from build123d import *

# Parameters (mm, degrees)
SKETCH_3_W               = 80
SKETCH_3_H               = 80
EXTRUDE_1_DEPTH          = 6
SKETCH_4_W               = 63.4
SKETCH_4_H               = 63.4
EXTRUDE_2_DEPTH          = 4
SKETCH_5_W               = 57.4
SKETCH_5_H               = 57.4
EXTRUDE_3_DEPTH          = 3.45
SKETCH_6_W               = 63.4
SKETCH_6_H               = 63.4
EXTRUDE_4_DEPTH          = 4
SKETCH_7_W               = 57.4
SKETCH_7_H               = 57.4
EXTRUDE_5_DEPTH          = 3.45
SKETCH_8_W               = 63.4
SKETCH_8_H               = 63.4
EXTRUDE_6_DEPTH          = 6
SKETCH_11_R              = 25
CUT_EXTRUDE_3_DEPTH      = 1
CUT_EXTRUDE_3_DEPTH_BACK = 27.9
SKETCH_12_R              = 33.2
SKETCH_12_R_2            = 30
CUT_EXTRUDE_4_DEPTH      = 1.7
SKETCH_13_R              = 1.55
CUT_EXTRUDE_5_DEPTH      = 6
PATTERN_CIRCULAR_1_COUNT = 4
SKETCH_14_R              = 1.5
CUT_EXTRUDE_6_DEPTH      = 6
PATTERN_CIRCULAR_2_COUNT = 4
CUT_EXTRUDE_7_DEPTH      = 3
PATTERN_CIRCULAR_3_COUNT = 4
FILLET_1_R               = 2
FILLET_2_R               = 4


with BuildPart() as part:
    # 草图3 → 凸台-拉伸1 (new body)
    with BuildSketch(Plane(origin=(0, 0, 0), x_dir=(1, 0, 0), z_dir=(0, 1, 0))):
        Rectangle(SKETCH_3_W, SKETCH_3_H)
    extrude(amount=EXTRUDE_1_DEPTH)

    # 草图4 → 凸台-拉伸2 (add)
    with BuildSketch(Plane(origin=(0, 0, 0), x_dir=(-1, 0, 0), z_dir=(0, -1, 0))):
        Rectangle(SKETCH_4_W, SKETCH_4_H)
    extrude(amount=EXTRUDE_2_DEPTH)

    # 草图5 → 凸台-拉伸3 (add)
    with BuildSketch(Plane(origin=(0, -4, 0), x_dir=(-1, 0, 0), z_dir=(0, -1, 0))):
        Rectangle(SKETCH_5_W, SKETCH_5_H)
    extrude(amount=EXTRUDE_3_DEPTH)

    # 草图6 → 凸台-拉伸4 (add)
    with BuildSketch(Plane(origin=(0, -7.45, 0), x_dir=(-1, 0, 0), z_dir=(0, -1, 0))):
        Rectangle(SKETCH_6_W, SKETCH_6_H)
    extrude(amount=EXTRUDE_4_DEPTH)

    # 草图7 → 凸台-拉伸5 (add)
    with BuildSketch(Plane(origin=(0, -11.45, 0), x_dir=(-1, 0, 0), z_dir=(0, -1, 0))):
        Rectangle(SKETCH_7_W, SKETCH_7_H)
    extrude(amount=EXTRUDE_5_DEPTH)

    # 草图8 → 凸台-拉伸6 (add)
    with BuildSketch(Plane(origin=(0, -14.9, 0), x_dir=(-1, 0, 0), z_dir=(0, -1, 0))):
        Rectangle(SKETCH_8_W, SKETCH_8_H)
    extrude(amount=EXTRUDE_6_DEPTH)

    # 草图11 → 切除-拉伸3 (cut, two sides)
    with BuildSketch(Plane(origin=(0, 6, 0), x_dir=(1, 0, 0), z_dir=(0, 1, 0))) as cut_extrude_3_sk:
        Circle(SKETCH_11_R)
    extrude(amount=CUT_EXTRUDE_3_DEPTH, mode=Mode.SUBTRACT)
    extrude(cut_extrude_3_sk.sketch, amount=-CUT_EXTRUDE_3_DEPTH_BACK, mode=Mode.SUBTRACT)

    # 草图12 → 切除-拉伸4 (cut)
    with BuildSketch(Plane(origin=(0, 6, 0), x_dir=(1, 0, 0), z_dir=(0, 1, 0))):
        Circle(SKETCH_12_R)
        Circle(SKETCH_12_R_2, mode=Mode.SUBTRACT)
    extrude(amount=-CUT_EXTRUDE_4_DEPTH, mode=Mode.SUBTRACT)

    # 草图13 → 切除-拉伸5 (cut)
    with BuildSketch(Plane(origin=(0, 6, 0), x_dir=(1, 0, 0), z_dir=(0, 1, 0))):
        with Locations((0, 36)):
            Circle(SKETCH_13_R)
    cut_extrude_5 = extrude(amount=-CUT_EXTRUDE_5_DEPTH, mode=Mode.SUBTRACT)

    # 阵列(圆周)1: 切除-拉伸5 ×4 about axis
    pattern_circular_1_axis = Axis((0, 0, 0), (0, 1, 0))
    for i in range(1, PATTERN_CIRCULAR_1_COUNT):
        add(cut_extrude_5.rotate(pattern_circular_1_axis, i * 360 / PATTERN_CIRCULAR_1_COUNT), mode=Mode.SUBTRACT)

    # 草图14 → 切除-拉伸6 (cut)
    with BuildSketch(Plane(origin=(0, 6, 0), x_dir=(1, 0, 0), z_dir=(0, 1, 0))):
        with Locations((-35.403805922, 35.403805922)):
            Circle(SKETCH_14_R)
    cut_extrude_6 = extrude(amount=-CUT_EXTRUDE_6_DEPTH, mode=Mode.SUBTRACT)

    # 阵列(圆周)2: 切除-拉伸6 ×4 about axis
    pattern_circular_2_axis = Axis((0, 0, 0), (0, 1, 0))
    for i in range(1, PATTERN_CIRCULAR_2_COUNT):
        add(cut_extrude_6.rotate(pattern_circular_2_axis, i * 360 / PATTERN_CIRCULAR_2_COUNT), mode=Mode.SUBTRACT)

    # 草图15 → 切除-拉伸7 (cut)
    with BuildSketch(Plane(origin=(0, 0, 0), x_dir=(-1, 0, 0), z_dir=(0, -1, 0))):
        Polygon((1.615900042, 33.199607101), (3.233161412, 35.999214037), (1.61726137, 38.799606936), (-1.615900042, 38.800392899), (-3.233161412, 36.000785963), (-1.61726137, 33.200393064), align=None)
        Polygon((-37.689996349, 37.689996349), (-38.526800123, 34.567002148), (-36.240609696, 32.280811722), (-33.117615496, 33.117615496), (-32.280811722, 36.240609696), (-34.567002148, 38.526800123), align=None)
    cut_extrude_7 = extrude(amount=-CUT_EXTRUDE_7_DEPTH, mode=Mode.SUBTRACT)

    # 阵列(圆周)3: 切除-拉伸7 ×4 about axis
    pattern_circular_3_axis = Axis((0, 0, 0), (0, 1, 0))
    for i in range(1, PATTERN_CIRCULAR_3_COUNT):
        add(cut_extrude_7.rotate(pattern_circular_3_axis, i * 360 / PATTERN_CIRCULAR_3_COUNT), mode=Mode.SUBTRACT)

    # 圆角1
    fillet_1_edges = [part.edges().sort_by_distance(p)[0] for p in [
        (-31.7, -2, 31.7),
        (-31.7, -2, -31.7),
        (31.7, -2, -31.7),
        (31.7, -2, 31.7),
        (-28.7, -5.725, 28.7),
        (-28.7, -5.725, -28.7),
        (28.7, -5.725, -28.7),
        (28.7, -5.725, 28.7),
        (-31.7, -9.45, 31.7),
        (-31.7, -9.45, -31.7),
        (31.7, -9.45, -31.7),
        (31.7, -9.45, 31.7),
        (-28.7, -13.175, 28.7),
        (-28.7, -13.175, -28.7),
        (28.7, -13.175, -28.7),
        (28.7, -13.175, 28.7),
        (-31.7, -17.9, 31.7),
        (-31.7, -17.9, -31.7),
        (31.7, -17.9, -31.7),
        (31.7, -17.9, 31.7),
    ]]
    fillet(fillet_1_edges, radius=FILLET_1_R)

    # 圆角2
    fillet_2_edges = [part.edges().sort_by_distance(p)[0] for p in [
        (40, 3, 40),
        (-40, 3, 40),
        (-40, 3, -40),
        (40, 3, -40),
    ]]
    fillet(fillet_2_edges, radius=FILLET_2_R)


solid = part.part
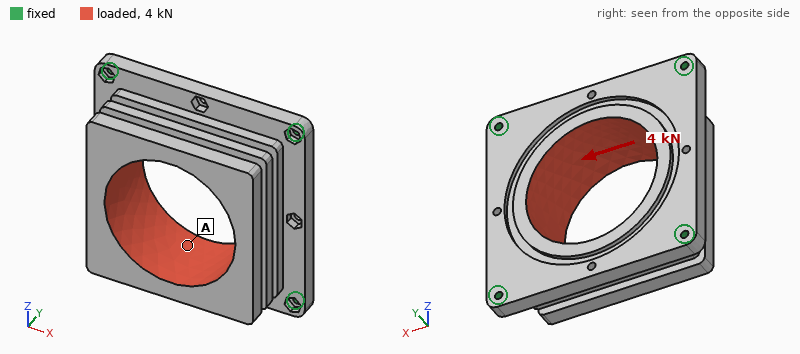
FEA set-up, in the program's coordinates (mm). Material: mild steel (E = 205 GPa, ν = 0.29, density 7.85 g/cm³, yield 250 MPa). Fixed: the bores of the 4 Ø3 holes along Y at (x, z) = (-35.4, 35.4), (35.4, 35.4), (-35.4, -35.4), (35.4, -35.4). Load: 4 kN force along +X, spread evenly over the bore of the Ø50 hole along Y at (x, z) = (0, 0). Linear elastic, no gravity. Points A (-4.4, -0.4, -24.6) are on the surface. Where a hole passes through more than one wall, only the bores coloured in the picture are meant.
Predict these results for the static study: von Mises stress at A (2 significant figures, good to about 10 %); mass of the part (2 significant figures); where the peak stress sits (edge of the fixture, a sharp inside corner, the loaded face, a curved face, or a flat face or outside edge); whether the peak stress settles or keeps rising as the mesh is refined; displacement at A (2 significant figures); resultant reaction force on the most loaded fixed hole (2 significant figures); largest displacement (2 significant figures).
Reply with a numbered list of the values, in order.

1. 6.7 MPa
2. 490 g
3. edge of the fixture
4. keeps rising
5. 1.8 µm
6. 1.1 kN
7. 4.8 µm
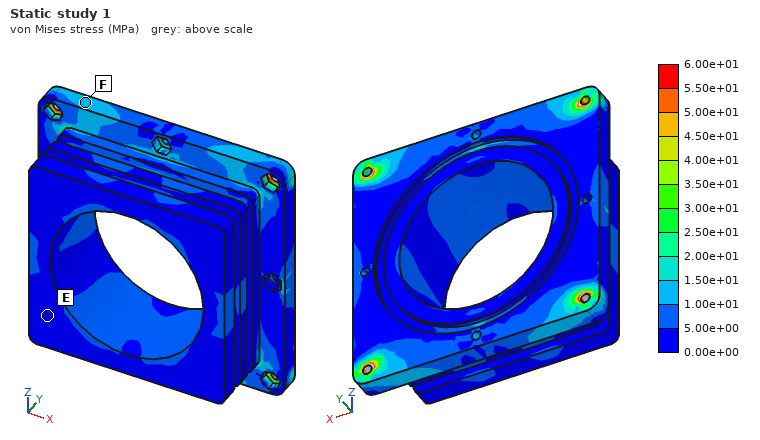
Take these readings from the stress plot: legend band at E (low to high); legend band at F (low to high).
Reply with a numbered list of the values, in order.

1. 0.00e+00 to 5.00e+00 MPa
2. 1.00e+01 to 1.50e+01 MPa
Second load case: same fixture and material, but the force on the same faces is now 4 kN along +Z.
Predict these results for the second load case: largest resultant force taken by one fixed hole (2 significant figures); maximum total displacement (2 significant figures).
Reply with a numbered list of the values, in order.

1. 1.1 kN
2. 4.8 µm
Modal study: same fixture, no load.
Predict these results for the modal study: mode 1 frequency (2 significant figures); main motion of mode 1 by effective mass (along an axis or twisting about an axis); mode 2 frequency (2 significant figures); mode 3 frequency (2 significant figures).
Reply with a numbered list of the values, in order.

1. 5400 Hz
2. along Y
3. 6700 Hz
4. 6700 Hz
